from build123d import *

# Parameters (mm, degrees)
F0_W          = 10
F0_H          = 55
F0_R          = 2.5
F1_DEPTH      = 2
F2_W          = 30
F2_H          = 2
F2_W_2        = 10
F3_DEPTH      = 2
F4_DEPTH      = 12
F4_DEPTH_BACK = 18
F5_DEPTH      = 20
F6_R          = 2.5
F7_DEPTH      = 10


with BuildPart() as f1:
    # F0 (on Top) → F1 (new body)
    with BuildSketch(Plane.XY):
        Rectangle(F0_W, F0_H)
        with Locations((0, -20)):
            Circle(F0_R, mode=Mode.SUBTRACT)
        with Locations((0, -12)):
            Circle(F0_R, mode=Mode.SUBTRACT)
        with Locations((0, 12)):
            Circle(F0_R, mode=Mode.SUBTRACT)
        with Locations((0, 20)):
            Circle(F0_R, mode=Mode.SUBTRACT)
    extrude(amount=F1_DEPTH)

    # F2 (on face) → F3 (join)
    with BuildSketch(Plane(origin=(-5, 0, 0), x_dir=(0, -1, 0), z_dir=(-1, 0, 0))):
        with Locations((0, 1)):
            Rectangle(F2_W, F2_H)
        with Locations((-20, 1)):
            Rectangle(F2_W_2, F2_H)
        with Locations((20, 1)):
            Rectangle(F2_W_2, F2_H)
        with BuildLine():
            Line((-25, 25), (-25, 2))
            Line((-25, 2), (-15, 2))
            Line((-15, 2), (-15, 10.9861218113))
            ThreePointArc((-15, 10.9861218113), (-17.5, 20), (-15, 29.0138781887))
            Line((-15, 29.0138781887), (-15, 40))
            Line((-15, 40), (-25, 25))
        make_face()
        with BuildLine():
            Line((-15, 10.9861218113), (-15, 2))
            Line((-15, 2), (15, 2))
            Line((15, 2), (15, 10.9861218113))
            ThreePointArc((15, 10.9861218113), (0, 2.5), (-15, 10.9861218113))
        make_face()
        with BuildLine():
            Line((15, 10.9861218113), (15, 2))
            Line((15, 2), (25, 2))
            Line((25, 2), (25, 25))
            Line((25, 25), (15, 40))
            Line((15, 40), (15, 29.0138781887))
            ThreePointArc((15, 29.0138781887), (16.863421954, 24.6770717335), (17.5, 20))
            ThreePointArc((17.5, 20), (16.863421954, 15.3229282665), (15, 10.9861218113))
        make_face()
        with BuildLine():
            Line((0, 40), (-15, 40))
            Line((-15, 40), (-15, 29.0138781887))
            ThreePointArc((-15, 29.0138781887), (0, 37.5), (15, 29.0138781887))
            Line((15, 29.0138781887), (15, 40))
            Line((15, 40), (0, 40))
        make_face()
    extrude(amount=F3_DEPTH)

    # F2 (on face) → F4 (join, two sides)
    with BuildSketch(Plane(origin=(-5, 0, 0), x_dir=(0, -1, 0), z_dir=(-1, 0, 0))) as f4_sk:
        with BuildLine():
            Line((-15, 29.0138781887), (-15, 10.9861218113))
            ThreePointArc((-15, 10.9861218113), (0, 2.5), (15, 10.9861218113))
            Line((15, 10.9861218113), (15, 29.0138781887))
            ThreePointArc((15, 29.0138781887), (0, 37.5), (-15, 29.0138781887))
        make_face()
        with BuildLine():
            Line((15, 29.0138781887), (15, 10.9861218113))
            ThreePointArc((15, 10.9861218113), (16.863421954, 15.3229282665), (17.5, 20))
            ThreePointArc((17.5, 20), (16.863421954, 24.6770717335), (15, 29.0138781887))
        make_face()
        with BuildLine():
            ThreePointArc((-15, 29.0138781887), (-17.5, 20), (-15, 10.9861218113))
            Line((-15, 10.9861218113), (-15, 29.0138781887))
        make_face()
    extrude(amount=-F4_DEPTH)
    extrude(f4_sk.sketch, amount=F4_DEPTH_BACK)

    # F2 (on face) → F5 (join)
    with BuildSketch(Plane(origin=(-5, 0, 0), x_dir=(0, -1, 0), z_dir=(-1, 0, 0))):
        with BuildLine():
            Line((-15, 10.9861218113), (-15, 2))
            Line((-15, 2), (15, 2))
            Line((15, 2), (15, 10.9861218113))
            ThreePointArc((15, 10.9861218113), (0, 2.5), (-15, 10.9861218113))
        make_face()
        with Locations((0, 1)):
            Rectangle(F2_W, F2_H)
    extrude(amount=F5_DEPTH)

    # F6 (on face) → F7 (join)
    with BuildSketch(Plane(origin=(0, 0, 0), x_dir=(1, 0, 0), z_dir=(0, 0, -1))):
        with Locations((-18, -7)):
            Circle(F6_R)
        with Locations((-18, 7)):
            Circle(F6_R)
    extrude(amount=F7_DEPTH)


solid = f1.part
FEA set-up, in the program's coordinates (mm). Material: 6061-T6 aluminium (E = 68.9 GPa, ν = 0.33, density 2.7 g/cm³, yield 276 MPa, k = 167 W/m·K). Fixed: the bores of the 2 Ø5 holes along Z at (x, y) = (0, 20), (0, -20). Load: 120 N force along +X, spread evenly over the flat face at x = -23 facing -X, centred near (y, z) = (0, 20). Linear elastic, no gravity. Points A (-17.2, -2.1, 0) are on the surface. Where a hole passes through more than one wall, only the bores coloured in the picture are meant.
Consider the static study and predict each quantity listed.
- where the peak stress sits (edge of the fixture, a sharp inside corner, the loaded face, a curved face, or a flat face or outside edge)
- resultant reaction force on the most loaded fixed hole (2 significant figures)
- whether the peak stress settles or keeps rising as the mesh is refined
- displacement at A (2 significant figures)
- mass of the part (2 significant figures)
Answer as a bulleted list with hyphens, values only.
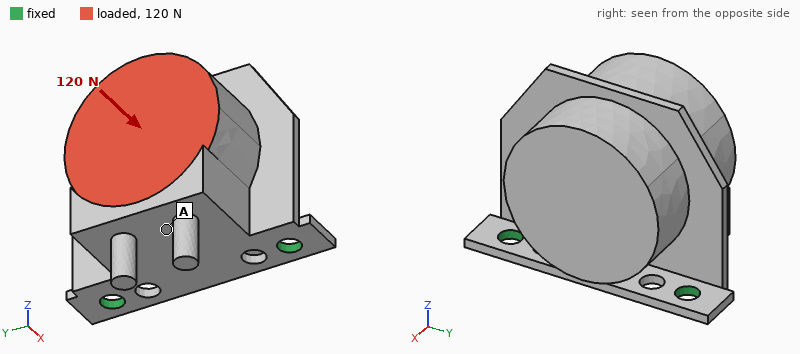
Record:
- edge of the fixture
- 60 N
- keeps rising
- 0.100 mm
- 94 g
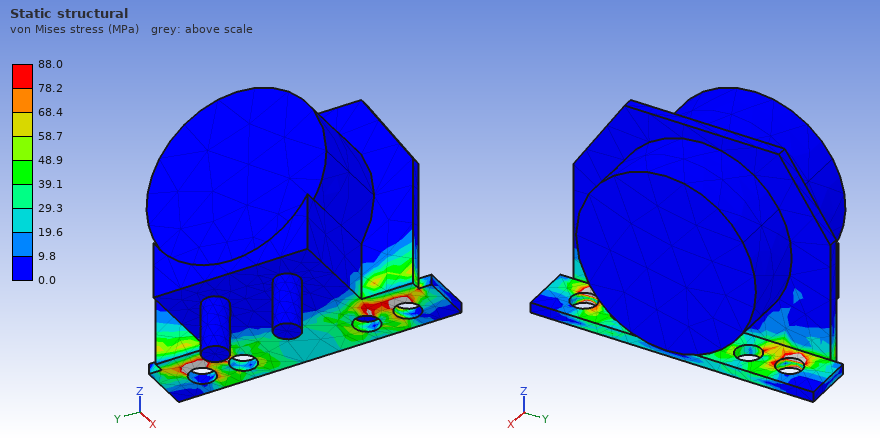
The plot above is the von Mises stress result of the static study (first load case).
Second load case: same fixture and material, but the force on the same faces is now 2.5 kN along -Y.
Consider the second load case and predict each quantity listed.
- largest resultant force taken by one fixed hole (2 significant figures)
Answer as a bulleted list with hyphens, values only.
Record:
- 2.2 kN
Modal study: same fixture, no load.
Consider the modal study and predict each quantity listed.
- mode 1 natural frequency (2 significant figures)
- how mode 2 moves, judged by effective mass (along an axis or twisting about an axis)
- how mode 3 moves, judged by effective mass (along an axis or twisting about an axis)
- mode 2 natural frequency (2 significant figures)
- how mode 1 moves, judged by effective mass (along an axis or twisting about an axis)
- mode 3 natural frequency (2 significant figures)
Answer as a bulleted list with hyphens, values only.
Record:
- 410 Hz
- along Y
- along Z
- 3300 Hz
- along X
- 4100 Hz
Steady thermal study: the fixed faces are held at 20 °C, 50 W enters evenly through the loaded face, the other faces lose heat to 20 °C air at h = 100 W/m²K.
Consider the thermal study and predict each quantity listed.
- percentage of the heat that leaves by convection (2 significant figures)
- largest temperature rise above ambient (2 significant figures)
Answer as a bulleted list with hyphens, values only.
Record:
- 43 %
- 36 K
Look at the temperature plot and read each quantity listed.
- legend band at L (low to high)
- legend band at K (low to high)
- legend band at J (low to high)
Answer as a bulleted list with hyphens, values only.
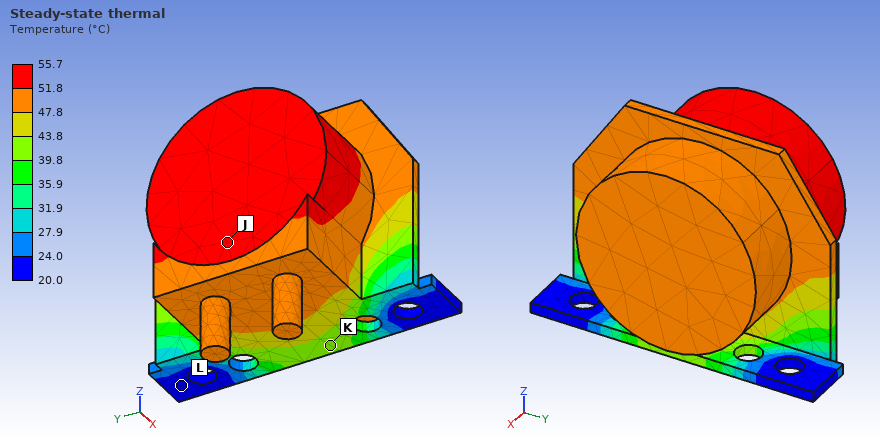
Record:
- 20.0 to 24.0 °C
- 39.8 to 43.8 °C
- 51.8 to 55.7 °C
